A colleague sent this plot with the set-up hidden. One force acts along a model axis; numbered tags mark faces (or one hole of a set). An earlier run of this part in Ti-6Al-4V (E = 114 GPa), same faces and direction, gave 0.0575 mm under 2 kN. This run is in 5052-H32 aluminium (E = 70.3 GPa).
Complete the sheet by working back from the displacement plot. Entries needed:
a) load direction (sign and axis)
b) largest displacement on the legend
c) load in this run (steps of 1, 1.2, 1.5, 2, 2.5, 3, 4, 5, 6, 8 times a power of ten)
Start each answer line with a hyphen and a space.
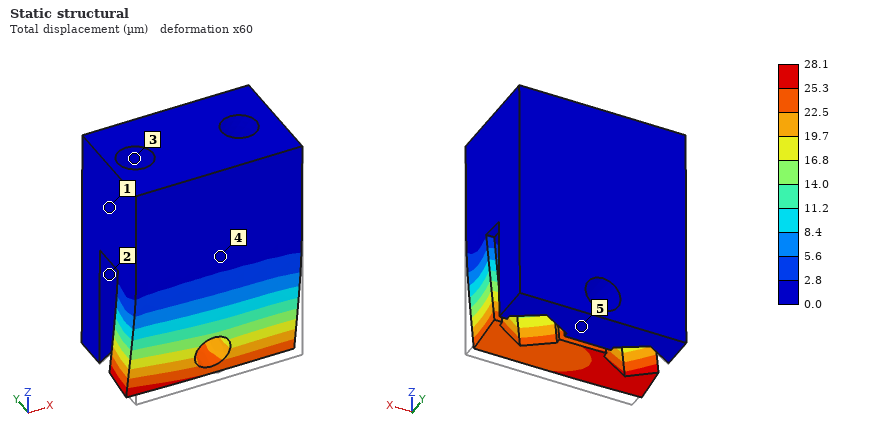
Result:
- +Y
- 28.1 µm
- 600 N
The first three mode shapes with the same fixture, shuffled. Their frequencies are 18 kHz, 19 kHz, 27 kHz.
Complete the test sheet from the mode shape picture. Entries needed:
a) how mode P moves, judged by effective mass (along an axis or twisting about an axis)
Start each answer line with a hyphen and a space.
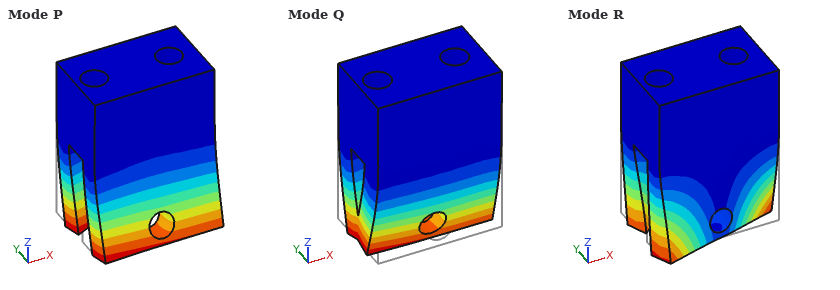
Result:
- along Y
